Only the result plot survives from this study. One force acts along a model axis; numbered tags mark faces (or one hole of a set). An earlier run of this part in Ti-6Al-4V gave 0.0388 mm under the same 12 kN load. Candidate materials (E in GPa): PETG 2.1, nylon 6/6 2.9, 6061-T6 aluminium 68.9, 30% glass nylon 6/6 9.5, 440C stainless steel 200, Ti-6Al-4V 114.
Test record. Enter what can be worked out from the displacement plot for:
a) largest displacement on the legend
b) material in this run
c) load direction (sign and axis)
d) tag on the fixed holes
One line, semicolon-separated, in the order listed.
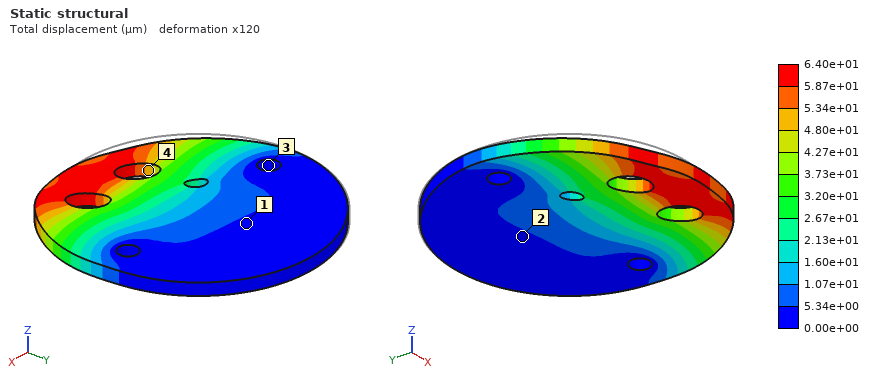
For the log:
6.40e+01 µm; 6061-T6 aluminium; +X; 3
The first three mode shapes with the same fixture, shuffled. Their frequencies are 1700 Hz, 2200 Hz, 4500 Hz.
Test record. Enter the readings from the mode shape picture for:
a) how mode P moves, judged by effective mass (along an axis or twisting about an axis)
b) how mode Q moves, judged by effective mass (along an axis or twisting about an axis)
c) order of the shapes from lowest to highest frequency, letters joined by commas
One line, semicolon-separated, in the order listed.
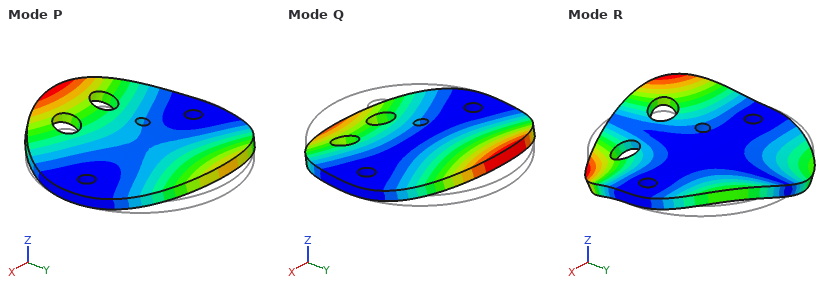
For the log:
along Z; twisting about X; Q, P, R
